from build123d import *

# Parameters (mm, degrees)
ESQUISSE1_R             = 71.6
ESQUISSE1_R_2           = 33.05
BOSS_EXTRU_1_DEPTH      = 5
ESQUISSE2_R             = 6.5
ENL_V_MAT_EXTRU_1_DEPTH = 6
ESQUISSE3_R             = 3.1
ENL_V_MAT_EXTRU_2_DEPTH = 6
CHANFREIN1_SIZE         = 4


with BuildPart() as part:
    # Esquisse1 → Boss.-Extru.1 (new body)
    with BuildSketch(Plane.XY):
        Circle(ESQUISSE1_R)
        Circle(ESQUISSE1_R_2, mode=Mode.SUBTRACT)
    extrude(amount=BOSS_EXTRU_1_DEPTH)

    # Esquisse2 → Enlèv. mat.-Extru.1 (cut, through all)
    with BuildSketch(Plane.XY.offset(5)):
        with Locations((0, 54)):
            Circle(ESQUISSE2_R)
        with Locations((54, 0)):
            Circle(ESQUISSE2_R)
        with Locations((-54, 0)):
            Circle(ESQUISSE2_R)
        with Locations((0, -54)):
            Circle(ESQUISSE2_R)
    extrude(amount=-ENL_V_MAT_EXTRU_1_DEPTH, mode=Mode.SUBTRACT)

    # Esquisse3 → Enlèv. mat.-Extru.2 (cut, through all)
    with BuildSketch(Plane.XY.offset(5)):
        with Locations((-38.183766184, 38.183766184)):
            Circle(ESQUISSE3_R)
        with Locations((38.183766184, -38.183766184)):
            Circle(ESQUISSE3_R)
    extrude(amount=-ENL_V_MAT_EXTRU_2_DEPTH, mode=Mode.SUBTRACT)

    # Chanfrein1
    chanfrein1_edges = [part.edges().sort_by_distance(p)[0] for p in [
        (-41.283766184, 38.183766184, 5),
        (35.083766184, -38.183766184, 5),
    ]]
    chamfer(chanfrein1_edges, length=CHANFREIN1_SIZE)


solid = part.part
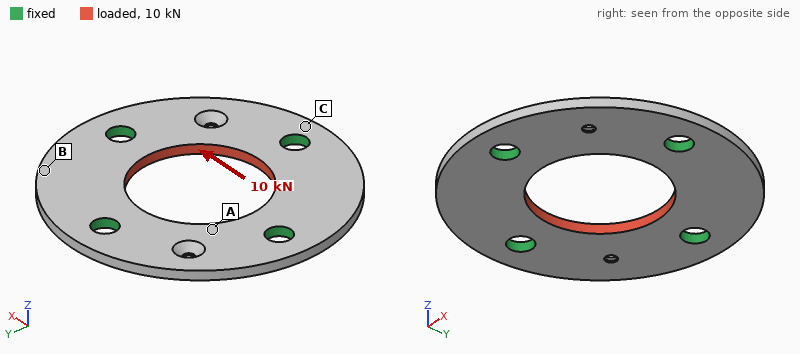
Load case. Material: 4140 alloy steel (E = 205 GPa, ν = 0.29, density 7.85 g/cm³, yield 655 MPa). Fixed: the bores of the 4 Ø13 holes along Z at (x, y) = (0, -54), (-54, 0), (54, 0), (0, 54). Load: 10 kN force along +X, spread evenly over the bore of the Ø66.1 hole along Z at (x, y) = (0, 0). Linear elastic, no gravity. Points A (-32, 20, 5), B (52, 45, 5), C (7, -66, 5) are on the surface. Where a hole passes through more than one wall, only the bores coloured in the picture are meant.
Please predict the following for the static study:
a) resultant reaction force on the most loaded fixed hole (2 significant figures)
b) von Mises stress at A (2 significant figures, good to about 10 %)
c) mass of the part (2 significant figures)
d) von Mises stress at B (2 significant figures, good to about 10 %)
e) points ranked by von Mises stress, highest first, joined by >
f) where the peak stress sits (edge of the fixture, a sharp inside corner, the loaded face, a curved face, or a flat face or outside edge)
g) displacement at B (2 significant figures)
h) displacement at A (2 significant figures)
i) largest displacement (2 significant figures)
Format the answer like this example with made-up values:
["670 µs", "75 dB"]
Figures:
["2.5 kN", "12 MPa", "470 g", "6.4 MPa", "A > B > C", "edge of the fixture", "1.8 µm", "2.3 µm", "2.9 µm"]
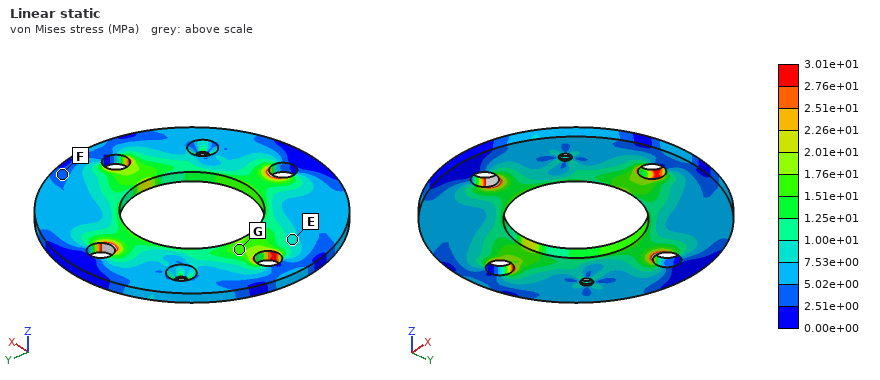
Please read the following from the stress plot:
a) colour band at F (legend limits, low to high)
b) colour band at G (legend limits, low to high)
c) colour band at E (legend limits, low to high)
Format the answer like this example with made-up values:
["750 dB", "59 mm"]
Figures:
["2.51e+00 to 5.02e+00 MPa", "1.51e+01 to 1.76e+01 MPa", "7.53e+00 to 1.00e+01 MPa"]
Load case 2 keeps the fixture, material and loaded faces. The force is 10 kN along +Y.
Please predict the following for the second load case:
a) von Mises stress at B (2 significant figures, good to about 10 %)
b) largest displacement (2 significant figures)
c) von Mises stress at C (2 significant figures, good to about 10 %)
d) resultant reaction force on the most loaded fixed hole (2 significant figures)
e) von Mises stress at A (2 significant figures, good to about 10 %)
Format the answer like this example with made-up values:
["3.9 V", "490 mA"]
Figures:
["6.5 MPa", "2.9 µm", "4.7 MPa", "2.5 kN", "8.5 MPa"]
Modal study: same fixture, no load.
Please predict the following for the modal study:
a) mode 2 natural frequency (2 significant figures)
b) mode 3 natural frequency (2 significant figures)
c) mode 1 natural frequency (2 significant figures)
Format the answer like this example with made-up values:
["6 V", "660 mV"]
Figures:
["3600 Hz", "3600 Hz", "3600 Hz"]
